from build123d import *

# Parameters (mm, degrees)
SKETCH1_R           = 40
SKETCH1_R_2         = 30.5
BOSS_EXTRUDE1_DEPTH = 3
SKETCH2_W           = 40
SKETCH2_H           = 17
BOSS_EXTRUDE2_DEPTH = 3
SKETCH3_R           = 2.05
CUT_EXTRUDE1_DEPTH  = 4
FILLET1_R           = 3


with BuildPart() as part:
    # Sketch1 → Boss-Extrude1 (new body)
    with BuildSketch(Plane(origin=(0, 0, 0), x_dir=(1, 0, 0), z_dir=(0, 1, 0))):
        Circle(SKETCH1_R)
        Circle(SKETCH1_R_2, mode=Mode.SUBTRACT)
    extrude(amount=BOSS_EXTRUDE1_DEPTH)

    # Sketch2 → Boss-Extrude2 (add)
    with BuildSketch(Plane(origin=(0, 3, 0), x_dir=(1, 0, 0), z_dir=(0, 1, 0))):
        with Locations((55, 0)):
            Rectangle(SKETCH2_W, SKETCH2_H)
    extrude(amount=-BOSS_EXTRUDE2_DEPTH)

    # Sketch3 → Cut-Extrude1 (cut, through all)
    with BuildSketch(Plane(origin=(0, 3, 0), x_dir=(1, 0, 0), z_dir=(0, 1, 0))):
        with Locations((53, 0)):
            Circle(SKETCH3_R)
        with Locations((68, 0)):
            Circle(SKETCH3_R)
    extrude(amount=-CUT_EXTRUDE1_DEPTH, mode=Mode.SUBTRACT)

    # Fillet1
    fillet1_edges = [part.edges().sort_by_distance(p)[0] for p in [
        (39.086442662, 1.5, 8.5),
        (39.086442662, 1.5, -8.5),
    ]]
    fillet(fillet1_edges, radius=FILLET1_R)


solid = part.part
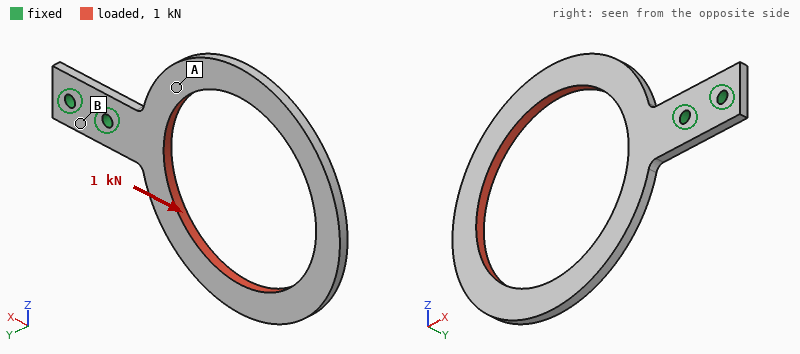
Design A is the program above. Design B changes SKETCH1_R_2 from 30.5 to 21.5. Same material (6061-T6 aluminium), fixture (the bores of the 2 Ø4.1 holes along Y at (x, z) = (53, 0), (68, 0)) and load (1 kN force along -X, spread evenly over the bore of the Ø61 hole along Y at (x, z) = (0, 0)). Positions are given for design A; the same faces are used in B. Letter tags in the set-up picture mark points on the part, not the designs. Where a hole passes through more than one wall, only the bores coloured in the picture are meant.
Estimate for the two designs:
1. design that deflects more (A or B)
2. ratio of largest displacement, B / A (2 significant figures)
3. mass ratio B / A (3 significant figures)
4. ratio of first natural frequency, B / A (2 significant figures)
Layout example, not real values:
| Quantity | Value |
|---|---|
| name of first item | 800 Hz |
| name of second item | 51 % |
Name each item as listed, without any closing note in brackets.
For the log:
| Quantity | Value |
|---|---|
| design that deflects more | A |
| ratio of largest displacement, B / A | 0.15 |
| mass ratio B / A | 1.55 |
| ratio of first natural frequency, B / A | 0.95 |
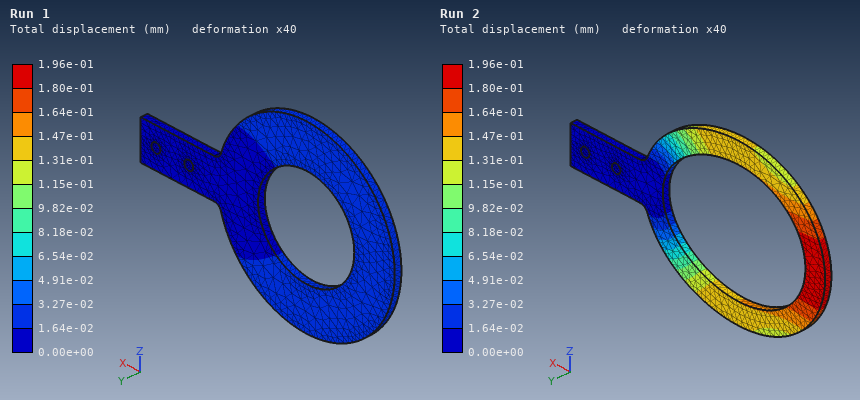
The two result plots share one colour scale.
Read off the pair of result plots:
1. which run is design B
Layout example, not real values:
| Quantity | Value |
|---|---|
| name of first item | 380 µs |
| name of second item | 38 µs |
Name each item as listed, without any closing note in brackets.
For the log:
| Quantity | Value |
|---|---|
| which run is design B | Run 1 |
